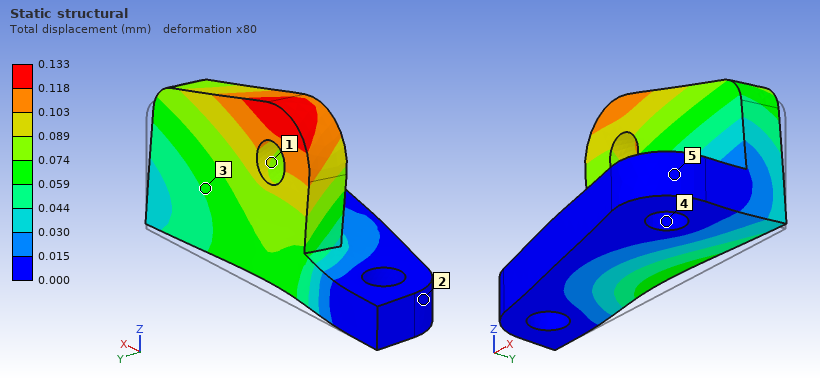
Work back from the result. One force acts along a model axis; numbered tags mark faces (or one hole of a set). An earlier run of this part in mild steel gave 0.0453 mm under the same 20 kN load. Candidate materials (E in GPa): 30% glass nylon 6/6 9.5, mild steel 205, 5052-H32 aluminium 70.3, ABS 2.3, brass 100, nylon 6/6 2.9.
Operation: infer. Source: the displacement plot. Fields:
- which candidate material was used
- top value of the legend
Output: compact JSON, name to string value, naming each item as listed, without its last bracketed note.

{"which candidate material was used": "5052-H32 aluminium", "top value of the legend": "0.133 mm"}
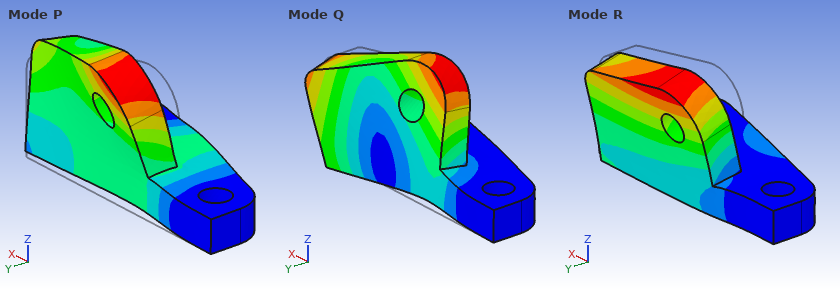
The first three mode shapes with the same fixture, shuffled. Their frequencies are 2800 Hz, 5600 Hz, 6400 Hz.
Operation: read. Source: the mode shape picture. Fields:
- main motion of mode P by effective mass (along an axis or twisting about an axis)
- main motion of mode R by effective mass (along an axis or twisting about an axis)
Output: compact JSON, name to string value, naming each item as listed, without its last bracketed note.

{"main motion of mode P by effective mass": "along Z", "main motion of mode R by effective mass": "along Y"}
